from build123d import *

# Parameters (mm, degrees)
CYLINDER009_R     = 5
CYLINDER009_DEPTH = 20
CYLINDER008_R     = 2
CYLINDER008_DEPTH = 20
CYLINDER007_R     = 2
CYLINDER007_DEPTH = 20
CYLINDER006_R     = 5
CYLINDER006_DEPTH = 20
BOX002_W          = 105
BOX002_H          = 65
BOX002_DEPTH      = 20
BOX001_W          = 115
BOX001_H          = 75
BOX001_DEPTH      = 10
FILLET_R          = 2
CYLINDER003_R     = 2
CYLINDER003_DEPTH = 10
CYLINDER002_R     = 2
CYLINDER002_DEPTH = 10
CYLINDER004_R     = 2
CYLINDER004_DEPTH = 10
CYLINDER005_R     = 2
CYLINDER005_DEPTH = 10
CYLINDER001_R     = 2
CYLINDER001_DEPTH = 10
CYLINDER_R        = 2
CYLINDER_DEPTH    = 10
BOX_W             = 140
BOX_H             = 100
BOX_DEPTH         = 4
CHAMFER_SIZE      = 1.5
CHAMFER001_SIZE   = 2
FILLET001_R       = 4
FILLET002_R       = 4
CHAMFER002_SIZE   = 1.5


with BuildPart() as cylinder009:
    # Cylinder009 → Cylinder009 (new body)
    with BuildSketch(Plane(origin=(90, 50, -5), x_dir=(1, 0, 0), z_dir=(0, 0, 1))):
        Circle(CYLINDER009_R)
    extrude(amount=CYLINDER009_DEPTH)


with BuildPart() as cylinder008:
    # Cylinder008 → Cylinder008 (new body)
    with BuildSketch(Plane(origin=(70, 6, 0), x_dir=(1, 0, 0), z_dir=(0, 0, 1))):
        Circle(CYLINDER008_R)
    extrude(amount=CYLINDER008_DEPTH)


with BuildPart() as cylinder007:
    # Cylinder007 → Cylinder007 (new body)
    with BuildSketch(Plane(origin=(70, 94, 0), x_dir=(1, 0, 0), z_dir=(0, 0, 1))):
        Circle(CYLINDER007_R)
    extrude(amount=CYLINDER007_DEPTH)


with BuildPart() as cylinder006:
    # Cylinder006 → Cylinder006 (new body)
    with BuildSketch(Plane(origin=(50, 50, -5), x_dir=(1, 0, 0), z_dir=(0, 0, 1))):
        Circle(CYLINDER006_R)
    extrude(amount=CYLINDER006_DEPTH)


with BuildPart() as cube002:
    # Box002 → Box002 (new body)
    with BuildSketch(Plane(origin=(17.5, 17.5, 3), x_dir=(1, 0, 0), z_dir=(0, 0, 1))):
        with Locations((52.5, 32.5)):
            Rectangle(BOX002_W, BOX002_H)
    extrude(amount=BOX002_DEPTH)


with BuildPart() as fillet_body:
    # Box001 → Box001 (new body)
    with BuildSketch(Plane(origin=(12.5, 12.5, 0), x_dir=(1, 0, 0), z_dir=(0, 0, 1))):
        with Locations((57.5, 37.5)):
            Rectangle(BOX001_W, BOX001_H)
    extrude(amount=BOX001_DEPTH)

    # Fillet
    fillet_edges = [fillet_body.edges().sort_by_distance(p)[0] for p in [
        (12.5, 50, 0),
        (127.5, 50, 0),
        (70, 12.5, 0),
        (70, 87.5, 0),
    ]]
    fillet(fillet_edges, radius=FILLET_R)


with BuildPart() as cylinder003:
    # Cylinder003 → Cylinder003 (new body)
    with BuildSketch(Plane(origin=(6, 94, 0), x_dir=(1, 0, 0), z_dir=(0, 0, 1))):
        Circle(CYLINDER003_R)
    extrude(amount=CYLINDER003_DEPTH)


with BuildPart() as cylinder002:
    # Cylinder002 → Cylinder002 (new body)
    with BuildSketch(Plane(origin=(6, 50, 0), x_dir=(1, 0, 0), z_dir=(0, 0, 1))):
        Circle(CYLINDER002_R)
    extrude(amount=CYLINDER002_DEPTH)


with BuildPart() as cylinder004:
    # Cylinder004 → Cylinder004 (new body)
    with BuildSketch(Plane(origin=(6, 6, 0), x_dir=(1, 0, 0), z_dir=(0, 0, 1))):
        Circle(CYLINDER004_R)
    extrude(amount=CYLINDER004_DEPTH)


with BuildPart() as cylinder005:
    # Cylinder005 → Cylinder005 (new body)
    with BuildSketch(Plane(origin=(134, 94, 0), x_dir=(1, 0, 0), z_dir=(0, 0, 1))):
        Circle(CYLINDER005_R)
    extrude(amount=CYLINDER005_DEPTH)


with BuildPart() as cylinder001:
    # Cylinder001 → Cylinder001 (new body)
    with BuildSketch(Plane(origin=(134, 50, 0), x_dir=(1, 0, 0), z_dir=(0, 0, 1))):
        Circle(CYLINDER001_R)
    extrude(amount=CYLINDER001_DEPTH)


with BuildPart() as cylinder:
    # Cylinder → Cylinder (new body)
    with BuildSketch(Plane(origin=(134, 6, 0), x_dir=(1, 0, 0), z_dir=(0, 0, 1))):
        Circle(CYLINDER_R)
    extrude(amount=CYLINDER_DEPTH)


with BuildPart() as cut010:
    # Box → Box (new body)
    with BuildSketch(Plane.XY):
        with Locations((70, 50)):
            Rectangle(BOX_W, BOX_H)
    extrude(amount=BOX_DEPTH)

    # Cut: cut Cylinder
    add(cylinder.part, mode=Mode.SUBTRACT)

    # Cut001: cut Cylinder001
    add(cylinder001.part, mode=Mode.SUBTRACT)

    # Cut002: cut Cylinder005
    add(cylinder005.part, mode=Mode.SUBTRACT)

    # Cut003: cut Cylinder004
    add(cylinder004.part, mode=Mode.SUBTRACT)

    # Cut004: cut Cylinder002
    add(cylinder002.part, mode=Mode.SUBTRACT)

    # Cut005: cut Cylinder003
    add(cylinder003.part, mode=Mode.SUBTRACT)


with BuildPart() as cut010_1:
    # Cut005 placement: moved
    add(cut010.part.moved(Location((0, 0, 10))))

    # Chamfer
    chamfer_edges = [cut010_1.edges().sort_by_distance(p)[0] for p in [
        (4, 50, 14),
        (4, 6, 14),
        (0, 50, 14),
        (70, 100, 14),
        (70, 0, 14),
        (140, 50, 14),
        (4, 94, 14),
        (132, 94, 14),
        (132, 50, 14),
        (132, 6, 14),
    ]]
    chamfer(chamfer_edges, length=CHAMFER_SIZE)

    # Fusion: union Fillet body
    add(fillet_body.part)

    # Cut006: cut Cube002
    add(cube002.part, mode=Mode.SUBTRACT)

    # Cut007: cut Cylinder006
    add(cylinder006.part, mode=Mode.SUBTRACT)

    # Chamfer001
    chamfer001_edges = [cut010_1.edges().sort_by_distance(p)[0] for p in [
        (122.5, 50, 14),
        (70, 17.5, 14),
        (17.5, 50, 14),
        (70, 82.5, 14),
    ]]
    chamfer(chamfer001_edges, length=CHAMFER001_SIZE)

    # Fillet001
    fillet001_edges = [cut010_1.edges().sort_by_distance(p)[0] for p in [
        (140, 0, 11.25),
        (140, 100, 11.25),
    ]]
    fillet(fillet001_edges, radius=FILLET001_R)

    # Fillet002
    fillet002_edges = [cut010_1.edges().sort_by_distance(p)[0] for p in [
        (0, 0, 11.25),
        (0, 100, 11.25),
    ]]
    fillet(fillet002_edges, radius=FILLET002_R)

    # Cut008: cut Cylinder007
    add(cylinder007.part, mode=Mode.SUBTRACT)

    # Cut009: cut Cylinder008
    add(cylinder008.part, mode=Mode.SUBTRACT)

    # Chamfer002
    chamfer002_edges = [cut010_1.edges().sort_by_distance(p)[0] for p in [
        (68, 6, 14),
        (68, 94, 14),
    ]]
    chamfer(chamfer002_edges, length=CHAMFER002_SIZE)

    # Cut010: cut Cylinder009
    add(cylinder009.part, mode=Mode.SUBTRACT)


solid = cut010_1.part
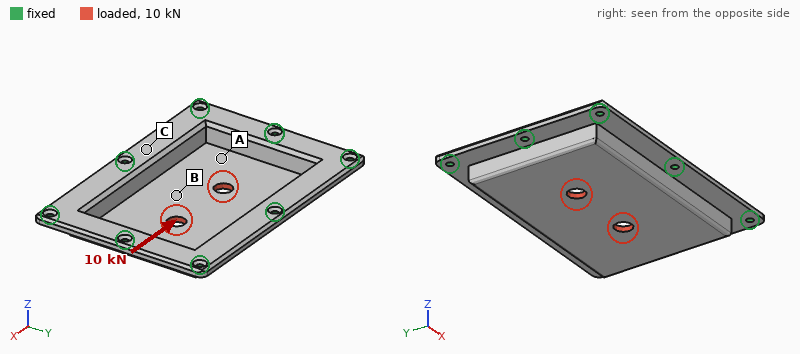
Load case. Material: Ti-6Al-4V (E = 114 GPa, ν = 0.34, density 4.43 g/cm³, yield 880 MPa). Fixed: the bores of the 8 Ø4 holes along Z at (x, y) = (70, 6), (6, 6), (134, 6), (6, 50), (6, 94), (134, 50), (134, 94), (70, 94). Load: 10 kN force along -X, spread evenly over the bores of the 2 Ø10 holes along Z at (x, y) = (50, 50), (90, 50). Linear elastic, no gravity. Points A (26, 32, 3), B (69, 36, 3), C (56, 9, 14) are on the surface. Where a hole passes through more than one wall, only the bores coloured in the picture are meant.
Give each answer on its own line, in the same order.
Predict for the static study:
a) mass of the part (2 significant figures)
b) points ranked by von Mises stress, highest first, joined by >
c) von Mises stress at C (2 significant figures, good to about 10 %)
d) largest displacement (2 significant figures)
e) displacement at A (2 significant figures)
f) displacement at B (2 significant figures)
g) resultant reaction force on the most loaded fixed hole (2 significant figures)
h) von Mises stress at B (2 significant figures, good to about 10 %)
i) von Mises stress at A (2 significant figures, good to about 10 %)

290 g
B > A > C
14 MPa
23 µm
13 µm
15 µm
2.2 kN
36 MPa
24 MPa
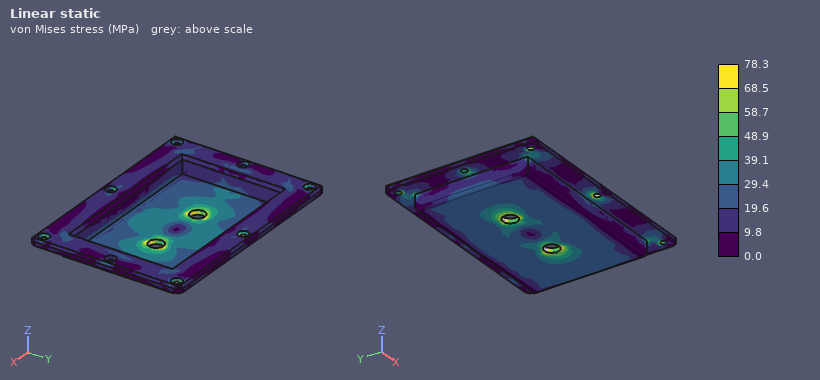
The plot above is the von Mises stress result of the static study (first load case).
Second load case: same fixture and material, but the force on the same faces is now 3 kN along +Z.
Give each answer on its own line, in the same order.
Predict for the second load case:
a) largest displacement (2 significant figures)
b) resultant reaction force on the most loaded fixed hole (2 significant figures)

0.26 mm
2.0 kN
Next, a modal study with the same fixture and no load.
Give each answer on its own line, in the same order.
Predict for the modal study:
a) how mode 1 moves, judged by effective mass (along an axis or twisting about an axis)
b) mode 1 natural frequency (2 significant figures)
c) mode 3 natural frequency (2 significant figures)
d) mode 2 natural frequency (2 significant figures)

along Z
3700 Hz
6200 Hz
5400 Hz
